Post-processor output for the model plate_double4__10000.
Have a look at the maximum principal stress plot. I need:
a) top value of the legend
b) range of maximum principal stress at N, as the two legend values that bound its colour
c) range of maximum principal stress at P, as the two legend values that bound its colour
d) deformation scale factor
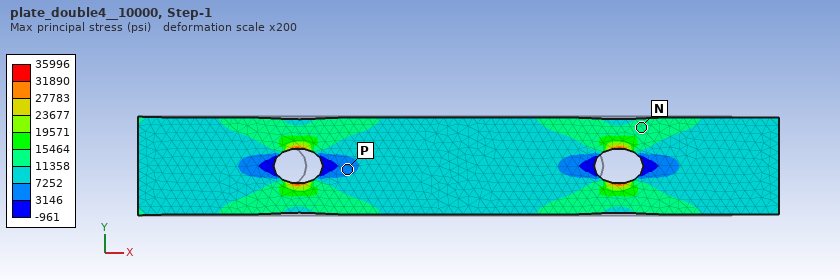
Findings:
35996 psi
11358 to 15464 psi
3146 to 7252 psi
200
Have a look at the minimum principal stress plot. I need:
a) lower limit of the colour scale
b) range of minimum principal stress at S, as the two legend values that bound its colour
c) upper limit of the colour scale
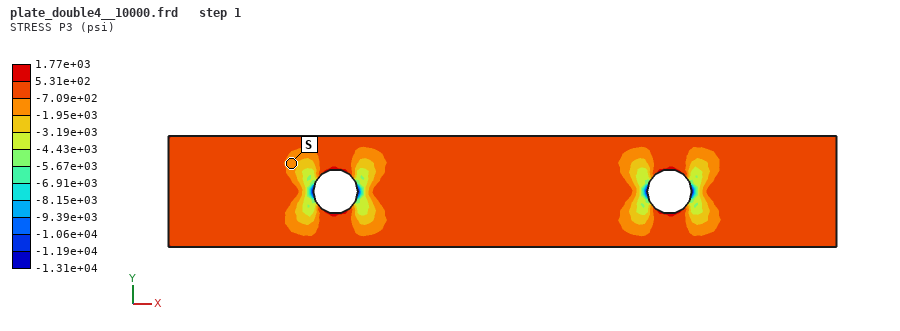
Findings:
-1.31e+04 psi
-1.95e+03 to -7.09e+02 psi
1.77e+03 psi
